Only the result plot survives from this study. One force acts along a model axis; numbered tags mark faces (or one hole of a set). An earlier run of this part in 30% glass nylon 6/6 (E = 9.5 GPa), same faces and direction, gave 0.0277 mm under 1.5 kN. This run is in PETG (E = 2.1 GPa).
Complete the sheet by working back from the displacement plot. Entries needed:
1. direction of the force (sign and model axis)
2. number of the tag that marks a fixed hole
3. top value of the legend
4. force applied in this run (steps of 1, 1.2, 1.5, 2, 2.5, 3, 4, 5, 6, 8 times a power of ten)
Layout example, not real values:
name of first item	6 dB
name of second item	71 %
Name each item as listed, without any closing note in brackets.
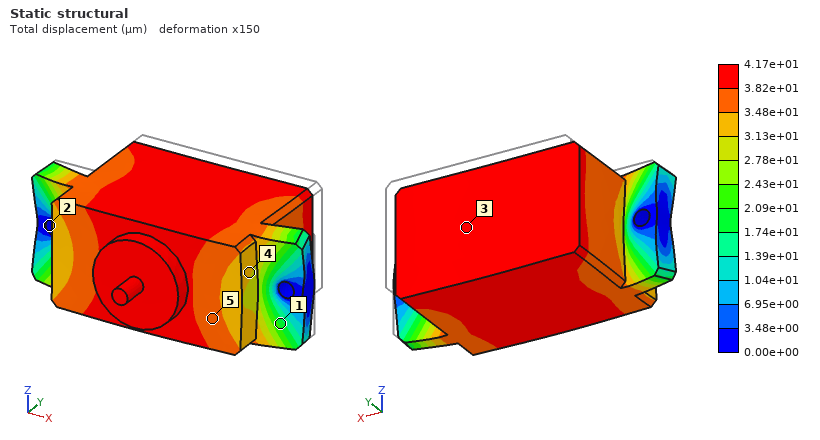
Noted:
direction of the force	-Y
number of the tag that marks a fixed hole	2
top value of the legend	4.17e+01 µm
force applied in this run	500 N
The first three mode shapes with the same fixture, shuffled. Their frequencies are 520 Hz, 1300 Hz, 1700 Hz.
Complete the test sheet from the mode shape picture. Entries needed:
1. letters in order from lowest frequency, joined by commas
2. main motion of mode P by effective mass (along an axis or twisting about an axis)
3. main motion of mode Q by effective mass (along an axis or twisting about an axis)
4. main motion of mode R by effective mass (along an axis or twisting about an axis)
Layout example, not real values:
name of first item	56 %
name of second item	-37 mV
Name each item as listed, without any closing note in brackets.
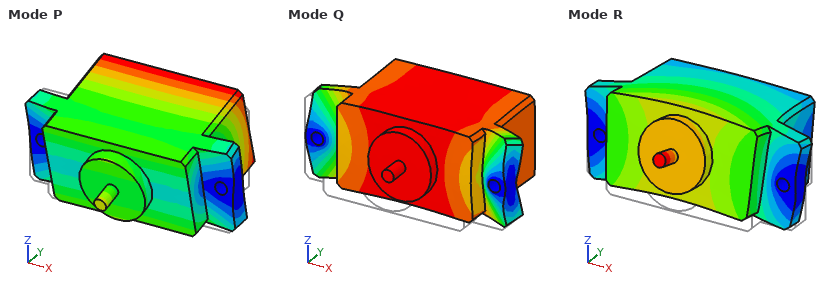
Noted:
letters in order from lowest frequency, joined by commas	P, Q, R
main motion of mode P by effective mass	along Z
main motion of mode Q by effective mass	along Y
main motion of mode R by effective mass	along Z
